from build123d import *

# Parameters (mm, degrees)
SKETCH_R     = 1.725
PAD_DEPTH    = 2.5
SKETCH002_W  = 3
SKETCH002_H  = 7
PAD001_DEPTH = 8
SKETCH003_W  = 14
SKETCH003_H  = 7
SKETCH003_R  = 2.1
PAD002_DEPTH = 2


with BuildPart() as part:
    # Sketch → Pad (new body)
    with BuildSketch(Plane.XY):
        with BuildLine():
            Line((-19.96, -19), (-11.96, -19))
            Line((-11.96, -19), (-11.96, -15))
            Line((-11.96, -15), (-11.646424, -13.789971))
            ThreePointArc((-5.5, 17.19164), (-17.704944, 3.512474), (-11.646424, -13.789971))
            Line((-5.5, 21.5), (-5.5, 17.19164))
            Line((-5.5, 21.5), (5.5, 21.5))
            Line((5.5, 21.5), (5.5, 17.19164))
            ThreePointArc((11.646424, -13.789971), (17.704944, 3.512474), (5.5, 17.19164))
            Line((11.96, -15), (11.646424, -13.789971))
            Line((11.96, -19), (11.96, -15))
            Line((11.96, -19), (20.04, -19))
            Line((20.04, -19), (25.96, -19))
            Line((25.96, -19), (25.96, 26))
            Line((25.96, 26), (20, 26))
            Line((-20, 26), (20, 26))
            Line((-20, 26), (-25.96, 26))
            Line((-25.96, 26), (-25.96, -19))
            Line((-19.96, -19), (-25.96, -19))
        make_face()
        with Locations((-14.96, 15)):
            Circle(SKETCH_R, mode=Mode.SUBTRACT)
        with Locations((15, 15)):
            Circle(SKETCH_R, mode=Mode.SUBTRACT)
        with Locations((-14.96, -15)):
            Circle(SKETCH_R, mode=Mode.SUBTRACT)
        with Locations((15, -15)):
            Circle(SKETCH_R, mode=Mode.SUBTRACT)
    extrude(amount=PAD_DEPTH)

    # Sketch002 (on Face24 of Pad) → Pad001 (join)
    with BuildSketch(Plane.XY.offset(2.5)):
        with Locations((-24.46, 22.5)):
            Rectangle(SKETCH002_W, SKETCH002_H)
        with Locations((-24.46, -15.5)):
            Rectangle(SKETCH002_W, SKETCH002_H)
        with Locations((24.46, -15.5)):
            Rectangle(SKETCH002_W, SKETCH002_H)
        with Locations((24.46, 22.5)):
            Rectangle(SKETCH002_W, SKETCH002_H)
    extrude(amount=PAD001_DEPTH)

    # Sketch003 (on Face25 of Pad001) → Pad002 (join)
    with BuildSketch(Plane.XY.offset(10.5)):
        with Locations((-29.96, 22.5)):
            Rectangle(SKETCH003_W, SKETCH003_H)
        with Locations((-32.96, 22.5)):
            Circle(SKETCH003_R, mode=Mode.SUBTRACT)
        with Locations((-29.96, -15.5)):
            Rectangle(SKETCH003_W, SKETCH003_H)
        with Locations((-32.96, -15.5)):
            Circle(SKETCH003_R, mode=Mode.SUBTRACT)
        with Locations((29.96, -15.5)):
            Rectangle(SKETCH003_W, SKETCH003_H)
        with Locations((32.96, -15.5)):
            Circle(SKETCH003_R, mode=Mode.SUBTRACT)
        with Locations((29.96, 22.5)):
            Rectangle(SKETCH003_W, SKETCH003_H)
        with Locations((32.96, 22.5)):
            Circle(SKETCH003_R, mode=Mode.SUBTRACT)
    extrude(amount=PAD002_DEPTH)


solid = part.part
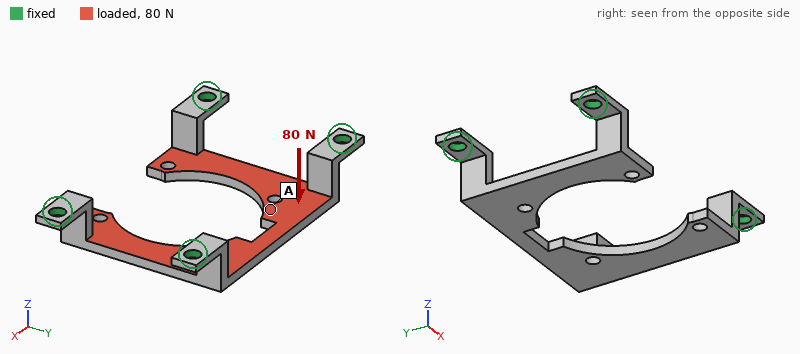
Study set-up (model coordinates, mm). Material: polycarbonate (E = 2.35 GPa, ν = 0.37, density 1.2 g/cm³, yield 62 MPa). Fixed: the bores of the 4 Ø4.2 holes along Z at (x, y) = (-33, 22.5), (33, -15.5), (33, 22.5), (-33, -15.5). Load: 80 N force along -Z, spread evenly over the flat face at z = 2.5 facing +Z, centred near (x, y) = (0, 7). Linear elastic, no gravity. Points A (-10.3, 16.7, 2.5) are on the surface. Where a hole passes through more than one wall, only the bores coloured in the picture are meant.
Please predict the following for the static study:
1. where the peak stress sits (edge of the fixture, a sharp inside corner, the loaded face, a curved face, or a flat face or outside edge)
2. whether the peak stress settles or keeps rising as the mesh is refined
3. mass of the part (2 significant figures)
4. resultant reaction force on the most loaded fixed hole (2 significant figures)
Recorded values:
edge of the fixture
keeps rising
5.1 g
37 N
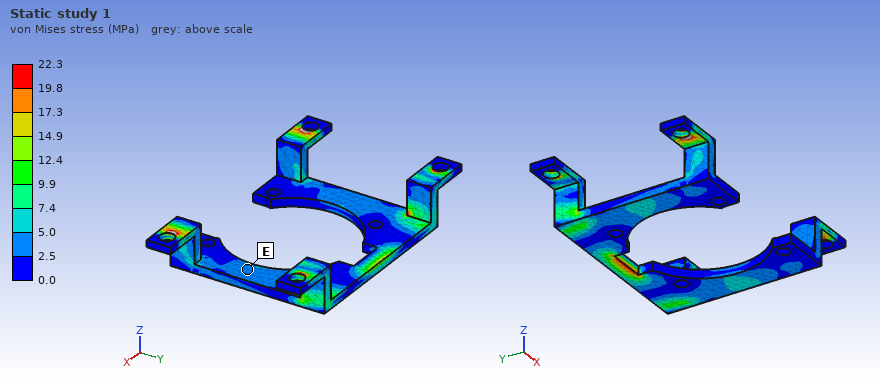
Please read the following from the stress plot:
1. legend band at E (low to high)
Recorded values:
2.5 to 5.0 MPa
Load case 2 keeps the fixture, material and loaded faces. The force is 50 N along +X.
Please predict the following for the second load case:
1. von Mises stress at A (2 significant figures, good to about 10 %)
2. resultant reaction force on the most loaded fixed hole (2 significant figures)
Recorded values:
3.8 MPa
18 N
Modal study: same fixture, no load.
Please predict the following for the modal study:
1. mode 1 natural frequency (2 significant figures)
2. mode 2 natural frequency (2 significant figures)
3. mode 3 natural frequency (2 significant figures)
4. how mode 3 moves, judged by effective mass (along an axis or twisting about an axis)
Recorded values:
820 Hz
840 Hz
1300 Hz
along Y
